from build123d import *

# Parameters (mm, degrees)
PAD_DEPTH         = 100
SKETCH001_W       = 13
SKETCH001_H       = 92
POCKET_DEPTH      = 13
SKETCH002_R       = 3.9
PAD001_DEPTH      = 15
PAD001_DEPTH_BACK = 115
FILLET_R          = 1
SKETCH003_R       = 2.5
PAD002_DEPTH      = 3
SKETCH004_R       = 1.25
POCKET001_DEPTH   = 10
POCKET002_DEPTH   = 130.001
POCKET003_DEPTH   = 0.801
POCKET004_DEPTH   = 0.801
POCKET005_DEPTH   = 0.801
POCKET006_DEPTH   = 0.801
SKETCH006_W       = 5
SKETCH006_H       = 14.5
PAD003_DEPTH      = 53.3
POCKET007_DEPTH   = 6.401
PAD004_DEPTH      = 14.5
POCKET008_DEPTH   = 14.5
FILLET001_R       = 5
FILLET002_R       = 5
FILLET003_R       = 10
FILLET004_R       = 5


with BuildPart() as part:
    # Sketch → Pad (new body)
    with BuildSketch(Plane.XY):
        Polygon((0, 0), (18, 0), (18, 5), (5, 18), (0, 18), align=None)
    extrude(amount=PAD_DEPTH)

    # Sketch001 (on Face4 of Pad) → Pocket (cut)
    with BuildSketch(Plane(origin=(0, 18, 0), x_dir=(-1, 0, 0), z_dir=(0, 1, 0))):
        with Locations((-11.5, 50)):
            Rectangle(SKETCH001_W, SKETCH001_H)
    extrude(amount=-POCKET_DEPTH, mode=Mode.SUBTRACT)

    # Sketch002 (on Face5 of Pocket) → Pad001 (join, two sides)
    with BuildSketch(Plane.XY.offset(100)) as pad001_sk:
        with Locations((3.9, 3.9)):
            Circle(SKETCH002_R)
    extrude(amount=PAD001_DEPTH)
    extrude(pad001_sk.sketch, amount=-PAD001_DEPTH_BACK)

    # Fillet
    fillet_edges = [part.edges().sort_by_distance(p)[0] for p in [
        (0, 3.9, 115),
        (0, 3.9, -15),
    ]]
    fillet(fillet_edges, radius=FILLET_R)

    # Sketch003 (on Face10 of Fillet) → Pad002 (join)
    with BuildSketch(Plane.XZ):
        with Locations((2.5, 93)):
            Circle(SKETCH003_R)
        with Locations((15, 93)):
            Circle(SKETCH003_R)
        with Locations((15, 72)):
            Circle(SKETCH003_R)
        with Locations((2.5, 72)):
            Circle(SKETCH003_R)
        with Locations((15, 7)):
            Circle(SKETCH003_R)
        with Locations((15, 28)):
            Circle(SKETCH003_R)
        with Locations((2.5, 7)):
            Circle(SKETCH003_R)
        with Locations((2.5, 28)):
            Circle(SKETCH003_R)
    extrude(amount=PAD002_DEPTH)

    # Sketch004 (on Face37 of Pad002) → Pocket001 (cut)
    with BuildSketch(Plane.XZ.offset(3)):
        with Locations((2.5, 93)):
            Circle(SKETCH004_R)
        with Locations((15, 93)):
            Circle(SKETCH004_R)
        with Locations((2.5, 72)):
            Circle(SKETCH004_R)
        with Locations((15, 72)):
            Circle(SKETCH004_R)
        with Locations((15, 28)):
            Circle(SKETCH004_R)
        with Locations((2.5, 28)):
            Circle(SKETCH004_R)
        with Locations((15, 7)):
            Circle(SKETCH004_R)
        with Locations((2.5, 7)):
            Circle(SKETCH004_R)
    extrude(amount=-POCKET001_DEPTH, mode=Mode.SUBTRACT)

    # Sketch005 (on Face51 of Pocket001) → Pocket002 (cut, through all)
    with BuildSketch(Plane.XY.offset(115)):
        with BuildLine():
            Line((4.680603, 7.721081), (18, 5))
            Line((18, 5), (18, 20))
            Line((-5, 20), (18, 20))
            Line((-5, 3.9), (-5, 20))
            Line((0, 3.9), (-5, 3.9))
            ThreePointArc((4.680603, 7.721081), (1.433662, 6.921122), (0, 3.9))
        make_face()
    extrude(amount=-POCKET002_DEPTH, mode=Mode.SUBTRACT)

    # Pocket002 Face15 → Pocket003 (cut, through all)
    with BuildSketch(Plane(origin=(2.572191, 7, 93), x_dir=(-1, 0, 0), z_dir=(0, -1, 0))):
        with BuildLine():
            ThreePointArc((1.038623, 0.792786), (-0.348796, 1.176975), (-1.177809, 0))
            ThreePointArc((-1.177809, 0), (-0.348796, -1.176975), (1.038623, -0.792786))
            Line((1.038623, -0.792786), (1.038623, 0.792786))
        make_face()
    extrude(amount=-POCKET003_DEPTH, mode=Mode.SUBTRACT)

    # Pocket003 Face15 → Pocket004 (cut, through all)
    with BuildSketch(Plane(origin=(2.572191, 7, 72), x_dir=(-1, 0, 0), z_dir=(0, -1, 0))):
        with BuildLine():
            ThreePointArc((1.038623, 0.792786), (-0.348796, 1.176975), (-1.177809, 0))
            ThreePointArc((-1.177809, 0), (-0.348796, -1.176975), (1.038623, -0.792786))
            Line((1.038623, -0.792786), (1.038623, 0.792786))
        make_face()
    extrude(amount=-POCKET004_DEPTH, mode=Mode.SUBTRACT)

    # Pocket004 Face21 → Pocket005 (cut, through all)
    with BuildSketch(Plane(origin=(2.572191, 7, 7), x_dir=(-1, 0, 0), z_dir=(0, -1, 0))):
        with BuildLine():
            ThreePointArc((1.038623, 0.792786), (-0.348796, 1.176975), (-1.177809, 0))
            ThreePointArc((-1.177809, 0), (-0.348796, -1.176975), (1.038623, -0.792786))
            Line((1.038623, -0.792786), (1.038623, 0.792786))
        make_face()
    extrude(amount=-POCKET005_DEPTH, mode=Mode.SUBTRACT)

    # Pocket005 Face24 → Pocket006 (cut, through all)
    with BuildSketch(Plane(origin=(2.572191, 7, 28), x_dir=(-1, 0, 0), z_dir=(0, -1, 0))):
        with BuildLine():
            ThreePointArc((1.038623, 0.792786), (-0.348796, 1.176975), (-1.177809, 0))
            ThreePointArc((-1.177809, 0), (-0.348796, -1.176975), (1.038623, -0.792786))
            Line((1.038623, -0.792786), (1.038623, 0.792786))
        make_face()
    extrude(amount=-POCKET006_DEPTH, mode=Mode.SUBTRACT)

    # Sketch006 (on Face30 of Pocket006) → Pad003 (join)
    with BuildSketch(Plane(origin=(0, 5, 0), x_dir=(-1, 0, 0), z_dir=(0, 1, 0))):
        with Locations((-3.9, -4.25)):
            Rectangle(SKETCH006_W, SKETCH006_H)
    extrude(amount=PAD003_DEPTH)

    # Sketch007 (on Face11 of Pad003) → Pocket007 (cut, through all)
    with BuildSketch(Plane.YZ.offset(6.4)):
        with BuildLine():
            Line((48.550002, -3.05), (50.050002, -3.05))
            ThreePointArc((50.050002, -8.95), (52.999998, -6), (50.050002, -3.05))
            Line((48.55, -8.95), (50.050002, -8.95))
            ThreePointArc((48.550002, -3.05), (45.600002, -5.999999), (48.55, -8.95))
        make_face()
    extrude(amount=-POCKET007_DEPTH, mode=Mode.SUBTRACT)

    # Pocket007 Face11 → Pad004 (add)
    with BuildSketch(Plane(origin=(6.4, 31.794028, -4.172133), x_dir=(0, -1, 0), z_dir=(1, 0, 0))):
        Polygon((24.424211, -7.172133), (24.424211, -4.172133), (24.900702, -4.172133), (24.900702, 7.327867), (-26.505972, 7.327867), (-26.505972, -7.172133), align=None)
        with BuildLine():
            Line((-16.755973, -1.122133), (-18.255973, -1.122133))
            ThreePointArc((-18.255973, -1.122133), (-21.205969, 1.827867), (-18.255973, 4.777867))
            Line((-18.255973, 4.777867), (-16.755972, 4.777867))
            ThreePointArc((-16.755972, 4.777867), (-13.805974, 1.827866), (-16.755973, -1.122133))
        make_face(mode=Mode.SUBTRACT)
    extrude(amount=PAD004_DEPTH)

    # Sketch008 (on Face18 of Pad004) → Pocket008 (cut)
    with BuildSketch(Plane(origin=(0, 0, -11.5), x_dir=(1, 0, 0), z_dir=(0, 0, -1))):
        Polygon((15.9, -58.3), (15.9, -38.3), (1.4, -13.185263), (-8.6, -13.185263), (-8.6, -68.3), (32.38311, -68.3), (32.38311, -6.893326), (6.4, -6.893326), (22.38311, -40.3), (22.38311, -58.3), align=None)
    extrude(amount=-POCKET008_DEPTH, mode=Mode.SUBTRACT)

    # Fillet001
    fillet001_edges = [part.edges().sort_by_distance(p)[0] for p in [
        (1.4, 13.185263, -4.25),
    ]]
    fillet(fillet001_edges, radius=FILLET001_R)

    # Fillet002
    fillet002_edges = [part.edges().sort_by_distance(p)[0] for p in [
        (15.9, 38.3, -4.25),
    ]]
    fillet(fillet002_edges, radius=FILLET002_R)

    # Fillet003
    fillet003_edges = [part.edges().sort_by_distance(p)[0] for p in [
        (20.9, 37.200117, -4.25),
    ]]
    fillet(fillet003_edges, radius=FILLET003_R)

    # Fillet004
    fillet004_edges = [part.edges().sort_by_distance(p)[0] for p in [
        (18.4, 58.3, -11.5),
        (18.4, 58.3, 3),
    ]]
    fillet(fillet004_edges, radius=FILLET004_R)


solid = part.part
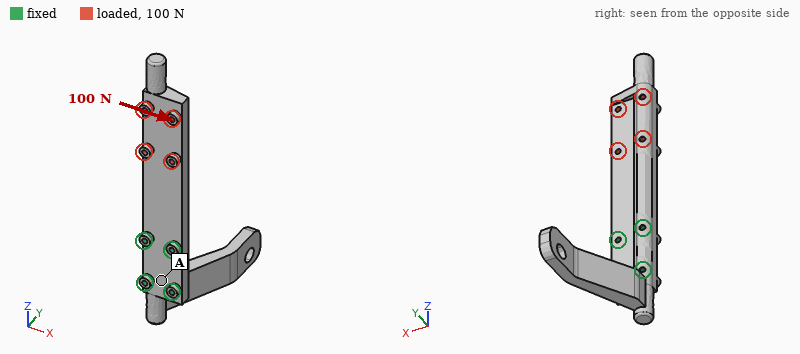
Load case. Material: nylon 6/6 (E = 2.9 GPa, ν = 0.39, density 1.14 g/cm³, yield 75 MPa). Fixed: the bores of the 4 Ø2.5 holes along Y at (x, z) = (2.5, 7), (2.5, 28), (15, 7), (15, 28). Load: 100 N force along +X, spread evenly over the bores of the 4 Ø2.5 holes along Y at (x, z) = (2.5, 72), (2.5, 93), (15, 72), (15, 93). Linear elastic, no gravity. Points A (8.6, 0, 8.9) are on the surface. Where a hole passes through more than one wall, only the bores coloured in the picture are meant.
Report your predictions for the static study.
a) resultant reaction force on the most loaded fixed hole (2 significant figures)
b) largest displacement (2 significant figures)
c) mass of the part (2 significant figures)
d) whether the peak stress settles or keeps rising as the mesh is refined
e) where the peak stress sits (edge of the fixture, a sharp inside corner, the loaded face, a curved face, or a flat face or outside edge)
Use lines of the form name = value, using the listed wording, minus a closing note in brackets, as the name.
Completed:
resultant reaction force on the most loaded fixed hole = 400 N
largest displacement = 1.6 mm
mass of the part = 19 g
whether the peak stress settles or keeps rising as the mesh is refined = keeps rising
where the peak stress sits = edge of the fixture
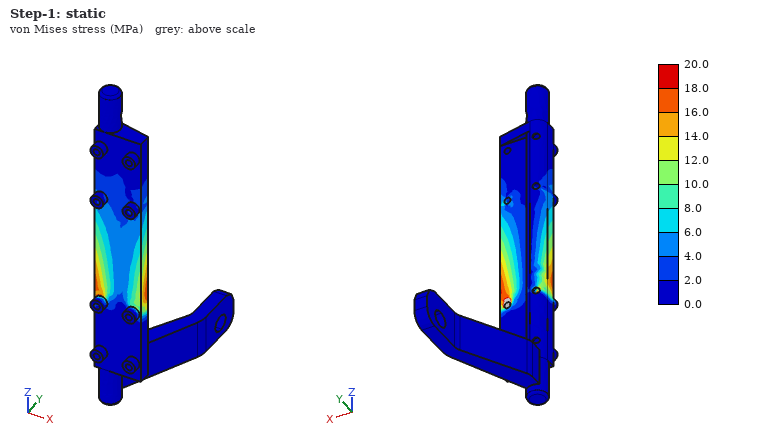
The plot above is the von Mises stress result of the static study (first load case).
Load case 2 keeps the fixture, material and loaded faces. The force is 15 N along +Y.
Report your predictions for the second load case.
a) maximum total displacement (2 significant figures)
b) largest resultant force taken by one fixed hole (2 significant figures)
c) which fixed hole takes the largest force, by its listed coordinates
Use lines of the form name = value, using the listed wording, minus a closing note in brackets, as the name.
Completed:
maximum total displacement = 1.5 mm
largest resultant force taken by one fixed hole = 18 N
which fixed hole takes the largest force, by its listed coordinates = (2.5, 28)
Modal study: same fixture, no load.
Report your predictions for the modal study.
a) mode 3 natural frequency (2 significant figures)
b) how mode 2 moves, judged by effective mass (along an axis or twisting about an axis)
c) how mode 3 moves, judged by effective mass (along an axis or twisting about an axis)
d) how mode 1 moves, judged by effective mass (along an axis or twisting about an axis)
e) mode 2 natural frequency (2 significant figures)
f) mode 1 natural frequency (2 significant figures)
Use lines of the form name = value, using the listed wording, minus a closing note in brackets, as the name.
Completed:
mode 3 natural frequency = 630 Hz
how mode 2 moves, judged by effective mass = along X
how mode 3 moves, judged by effective mass = along Z
how mode 1 moves, judged by effective mass = along Y
mode 2 natural frequency = 460 Hz
mode 1 natural frequency = 250 Hz
